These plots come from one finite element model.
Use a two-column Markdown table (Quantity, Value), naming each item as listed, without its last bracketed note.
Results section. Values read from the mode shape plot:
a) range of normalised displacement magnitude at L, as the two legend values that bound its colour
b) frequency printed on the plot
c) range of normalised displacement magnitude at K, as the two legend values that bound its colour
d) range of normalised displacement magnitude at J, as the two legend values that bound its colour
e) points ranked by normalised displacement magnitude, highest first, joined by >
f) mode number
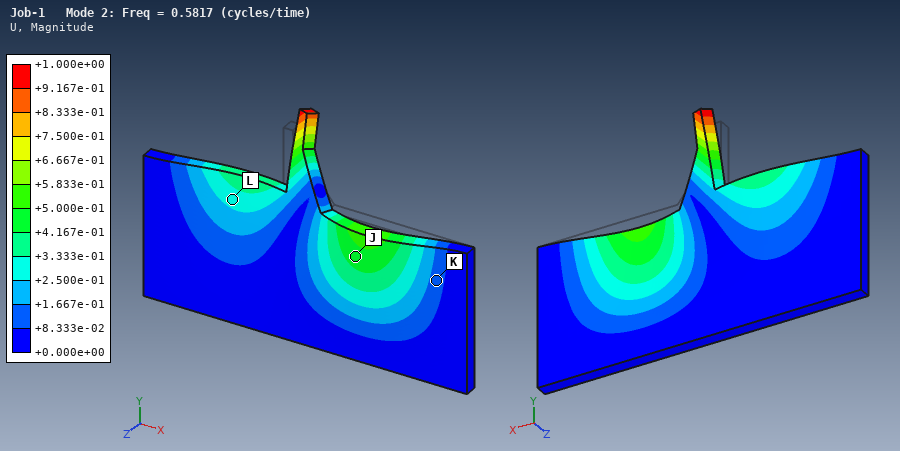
| Quantity | Value |
|---|---|
| range of normalised displacement magnitude at L, as the two legend values that bound its colour | +2.500e-01 to +3.333e-01 |
| frequency printed on the plot | 0.5817 |
| range of normalised displacement magnitude at K, as the two legend values that bound its colour | +8.333e-02 to +1.667e-01 |
| range of normalised displacement magnitude at J, as the two legend values that bound its colour | +4.167e-01 to +5.000e-01 |
| points ranked by normalised displacement magnitude, highest first, joined by > | J > L > K |
| mode number | 2 |
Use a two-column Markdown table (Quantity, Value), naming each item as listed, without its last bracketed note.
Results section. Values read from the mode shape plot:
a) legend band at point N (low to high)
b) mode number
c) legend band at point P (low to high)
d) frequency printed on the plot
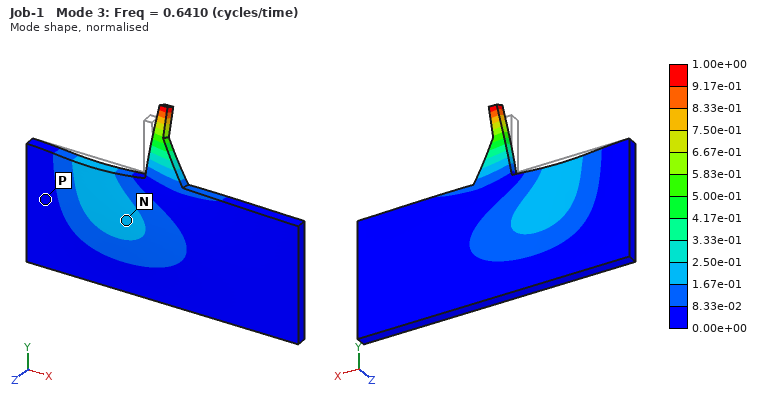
| Quantity | Value |
|---|---|
| legend band at point N | 1.67e-01 to 2.50e-01 |
| mode number | 3 |
| legend band at point P | 0.00e+00 to 8.33e-02 |
| frequency printed on the plot | 0.6410 |
